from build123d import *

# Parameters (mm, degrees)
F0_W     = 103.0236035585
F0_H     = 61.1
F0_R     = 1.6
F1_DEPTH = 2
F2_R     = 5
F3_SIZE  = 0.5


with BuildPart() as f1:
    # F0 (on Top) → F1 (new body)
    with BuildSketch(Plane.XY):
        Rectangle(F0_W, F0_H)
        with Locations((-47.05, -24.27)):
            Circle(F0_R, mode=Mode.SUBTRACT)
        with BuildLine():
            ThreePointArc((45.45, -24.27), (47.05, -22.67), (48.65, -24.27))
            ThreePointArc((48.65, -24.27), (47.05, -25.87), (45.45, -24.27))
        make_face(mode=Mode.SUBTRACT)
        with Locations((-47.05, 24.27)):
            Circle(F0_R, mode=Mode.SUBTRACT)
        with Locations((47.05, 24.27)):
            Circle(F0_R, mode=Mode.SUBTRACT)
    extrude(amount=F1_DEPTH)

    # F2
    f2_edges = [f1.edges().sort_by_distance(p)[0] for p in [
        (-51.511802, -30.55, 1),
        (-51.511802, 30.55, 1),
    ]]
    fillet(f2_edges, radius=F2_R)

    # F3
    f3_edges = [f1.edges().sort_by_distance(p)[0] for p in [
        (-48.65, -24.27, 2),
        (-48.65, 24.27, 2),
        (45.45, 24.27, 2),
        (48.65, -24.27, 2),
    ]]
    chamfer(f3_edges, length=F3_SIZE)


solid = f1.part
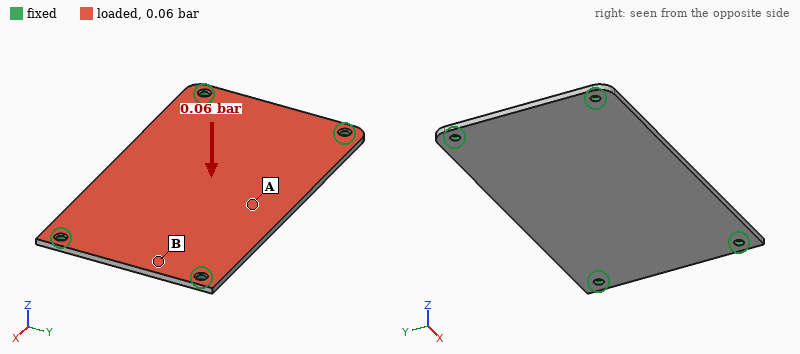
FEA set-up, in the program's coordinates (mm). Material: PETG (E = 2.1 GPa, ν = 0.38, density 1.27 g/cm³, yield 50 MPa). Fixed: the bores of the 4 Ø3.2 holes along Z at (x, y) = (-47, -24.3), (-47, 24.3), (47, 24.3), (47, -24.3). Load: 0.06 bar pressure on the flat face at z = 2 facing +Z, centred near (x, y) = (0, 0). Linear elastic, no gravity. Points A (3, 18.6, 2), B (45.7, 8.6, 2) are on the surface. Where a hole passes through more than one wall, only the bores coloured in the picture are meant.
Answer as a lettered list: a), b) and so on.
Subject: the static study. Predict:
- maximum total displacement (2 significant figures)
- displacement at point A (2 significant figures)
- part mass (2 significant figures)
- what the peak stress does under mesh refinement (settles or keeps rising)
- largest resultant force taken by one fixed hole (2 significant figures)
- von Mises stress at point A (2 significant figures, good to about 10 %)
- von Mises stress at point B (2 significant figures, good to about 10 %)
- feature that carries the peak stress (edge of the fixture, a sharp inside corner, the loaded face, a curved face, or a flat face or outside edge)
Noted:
a) 1.2 mm
b) 1.1 mm
c) 16 g
d) keeps rising
e) 9.9 N
f) 3.7 MPa
g) 1.7 MPa
h) edge of the fixture
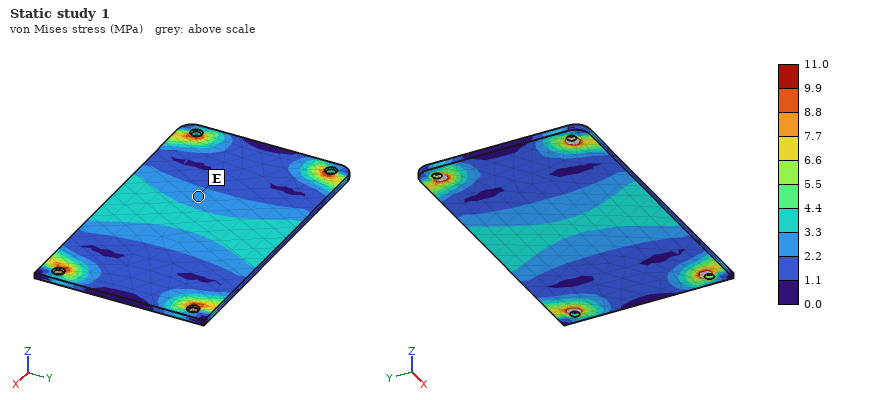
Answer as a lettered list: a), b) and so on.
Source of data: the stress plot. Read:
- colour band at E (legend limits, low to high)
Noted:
a) 2.2 to 3.3 MPa
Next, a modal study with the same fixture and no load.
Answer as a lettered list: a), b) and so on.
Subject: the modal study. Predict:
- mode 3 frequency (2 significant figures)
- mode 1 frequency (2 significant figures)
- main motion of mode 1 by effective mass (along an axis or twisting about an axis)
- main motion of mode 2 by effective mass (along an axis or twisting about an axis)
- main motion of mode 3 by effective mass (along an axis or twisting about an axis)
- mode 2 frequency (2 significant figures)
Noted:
a) 710 Hz
b) 260 Hz
c) along Z
d) twisting about X
e) twisting about Y
f) 420 Hz
